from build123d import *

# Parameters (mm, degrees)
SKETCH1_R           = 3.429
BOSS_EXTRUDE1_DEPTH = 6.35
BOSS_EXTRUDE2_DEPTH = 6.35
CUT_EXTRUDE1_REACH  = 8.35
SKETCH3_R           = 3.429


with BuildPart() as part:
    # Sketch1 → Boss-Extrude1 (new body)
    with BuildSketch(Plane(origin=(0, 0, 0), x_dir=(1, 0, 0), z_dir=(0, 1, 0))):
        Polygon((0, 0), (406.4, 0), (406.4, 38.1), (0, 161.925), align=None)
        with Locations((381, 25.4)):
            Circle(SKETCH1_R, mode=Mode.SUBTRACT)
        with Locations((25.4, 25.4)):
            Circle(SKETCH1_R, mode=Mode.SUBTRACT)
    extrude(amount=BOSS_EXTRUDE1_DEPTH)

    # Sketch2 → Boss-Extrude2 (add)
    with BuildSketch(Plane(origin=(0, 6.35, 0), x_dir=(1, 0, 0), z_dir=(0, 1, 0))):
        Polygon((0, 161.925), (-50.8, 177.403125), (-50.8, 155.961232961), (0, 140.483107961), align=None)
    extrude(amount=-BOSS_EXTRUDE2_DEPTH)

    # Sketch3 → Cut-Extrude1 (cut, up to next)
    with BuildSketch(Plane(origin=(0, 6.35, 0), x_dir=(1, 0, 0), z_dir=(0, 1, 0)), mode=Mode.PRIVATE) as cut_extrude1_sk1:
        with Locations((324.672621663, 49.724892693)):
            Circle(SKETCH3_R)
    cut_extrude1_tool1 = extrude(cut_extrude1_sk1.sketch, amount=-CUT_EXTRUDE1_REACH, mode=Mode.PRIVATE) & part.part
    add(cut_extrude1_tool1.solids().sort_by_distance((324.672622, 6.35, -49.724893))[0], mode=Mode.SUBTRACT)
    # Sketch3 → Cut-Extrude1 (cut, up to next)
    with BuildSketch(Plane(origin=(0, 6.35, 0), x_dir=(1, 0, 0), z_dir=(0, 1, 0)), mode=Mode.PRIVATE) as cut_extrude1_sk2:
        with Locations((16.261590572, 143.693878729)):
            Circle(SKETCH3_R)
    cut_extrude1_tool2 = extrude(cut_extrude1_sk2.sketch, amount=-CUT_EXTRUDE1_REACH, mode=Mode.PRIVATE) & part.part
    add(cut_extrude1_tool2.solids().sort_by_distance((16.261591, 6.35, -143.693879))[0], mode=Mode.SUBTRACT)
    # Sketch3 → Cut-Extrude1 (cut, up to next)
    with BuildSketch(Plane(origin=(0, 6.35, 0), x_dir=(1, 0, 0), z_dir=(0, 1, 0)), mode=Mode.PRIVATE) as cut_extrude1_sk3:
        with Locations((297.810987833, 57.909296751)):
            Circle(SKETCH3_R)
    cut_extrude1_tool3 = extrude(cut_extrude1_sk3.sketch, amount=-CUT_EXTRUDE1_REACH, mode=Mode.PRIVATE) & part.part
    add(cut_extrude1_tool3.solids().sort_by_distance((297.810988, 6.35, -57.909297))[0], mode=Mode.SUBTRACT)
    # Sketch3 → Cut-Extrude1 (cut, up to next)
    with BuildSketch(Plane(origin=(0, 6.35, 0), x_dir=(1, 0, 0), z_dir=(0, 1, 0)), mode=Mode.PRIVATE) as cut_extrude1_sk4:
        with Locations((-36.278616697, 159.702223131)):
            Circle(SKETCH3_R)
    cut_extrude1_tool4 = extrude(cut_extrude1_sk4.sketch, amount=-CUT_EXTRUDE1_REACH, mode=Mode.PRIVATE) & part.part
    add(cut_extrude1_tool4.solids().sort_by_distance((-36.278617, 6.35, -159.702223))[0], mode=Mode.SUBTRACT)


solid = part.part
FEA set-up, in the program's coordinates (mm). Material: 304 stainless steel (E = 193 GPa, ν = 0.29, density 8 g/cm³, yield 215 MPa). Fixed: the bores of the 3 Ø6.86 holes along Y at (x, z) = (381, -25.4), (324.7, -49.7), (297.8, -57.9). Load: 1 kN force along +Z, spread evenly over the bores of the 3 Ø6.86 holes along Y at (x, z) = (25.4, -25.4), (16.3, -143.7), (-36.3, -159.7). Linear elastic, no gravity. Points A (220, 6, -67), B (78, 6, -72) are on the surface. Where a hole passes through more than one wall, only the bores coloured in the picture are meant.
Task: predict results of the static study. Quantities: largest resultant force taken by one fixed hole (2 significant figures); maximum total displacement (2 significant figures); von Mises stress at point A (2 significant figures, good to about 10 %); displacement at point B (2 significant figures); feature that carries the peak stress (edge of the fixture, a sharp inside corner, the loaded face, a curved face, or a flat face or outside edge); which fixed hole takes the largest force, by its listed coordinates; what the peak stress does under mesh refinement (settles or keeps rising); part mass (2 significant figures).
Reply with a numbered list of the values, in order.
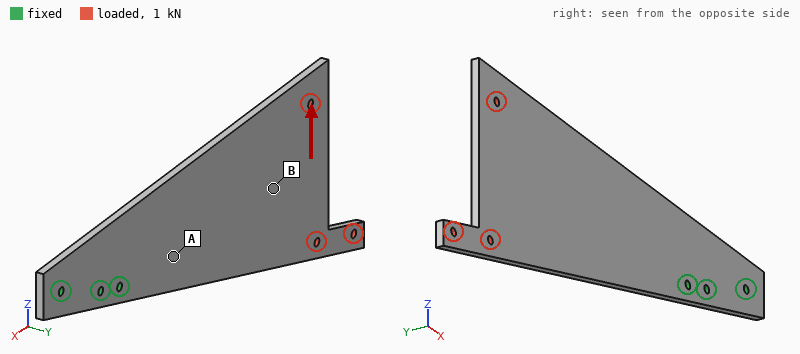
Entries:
1. 6.4 kN
2. 0.31 mm
3. 11 MPa
4. 0.15 mm
5. edge of the fixture
6. (297.8, -57.9)
7. keeps rising
8. 2.1 kg
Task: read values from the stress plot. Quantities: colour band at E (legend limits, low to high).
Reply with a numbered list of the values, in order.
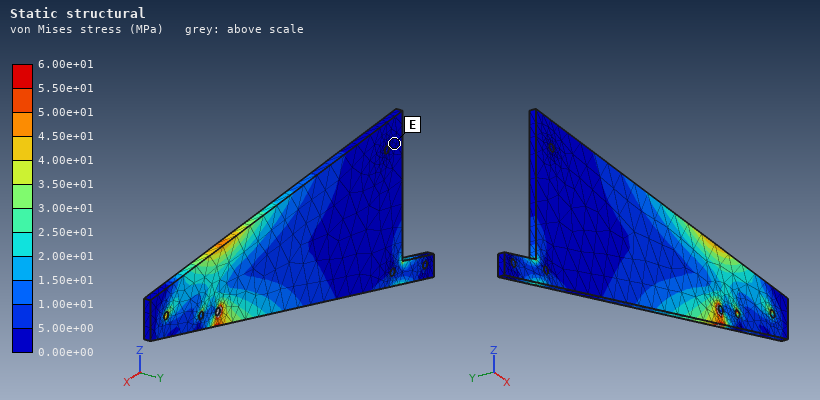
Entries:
1. 0.00e+00 to 5.00e+00 MPa
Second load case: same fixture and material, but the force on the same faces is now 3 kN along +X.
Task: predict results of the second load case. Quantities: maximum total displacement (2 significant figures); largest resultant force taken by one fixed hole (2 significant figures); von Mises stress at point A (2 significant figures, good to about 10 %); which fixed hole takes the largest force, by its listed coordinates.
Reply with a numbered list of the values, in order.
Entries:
1. 0.24 mm
2. 5.4 kN
3. 14 MPa
4. (297.8, -57.9)
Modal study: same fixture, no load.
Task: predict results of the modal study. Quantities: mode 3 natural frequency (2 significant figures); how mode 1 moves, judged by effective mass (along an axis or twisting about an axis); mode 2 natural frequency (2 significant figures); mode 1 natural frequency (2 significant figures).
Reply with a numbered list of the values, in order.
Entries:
1. 300 Hz
2. along Y
3. 170 Hz
4. 40 Hz
